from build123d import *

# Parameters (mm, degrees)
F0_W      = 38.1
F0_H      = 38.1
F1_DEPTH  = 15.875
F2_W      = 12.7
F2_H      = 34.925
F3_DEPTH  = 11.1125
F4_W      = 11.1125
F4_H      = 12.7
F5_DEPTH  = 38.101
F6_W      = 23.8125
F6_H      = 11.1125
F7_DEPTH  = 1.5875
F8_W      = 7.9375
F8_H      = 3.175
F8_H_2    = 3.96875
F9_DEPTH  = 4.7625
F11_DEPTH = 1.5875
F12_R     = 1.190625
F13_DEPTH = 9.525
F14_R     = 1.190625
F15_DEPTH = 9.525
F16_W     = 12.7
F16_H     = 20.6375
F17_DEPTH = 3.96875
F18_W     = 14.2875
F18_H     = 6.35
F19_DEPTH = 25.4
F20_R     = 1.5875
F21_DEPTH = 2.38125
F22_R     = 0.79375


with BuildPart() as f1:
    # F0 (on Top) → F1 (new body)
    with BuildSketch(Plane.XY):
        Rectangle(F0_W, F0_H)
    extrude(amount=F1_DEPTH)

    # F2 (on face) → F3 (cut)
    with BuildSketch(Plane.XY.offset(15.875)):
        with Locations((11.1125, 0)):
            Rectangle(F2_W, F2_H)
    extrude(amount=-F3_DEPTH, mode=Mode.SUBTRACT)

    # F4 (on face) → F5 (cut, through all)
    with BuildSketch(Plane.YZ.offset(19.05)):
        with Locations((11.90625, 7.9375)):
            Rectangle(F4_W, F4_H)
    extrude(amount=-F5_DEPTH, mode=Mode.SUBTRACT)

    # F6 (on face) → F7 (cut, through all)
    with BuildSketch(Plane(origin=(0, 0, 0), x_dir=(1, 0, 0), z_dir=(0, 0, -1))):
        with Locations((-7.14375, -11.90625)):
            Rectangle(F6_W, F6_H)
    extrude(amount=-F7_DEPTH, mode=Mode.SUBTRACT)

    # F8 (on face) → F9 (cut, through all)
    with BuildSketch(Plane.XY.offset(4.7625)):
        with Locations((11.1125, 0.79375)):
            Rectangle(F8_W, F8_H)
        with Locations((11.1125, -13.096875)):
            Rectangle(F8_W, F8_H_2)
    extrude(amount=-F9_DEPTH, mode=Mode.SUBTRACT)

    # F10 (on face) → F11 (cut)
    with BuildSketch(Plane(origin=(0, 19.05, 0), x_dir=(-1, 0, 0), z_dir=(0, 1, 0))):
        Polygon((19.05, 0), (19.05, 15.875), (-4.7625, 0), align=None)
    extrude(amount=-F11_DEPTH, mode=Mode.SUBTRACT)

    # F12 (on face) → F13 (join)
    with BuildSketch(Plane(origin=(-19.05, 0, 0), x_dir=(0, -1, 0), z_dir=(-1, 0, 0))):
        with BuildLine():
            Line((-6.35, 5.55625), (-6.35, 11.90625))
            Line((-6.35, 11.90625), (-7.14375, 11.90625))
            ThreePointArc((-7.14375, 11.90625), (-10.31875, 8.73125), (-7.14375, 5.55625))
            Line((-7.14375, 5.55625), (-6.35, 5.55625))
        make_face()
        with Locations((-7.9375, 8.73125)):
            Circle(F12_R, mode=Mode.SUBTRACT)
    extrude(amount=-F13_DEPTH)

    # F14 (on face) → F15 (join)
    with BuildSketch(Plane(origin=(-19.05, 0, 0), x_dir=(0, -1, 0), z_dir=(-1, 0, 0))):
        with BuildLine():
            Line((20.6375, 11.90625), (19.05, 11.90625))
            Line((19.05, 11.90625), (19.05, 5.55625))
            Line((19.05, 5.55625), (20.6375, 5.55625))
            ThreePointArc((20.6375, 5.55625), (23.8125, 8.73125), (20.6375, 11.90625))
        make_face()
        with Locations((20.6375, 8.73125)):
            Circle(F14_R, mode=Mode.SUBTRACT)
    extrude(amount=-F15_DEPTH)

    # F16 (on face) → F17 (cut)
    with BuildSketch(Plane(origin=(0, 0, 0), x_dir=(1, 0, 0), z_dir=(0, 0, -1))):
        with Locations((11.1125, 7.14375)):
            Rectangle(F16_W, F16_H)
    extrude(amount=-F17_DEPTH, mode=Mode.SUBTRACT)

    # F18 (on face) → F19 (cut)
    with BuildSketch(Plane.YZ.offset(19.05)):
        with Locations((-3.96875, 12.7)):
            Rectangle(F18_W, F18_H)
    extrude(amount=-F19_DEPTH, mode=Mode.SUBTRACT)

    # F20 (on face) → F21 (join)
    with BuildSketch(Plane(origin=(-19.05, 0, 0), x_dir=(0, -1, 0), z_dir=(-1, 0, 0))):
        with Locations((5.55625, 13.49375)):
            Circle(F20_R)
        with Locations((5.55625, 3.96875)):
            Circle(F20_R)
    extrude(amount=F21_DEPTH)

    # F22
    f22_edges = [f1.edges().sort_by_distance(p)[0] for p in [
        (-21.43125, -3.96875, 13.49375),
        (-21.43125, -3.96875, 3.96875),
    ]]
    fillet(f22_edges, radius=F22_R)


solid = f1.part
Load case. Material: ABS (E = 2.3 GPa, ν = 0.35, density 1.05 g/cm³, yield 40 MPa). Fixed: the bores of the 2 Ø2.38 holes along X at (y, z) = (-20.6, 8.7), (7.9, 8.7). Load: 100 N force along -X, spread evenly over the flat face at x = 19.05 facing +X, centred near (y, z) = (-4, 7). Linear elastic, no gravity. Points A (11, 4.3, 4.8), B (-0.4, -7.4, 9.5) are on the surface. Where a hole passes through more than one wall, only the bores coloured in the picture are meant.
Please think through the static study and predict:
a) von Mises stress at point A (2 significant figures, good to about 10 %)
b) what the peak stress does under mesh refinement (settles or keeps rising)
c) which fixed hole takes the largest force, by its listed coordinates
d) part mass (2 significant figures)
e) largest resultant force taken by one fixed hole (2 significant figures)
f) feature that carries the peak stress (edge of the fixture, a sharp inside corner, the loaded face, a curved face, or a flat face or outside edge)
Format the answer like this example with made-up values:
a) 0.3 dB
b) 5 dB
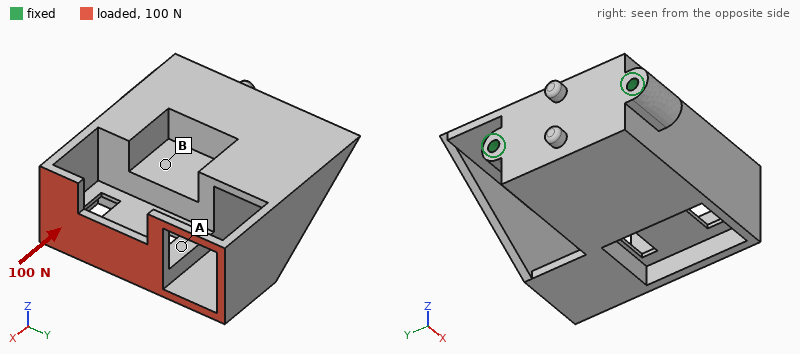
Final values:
a) 5.2 MPa
b) keeps rising
c) (7.9, 8.7)
d) 12 g
e) 61 N
f) a sharp inside corner
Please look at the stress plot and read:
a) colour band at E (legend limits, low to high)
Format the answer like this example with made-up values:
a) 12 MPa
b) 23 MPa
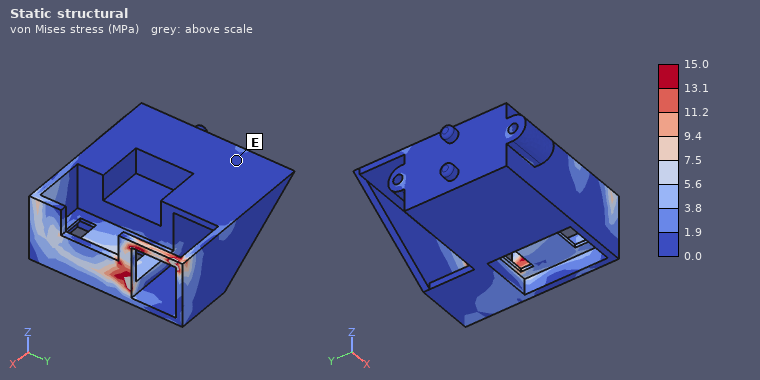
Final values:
a) 0.0 to 1.9 MPa
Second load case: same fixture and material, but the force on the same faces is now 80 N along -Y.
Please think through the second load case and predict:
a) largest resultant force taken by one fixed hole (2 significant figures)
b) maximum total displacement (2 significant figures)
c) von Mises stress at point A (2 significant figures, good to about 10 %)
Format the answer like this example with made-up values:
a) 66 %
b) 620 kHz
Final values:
a) 100 N
b) 0.40 mm
c) 5.6 MPa
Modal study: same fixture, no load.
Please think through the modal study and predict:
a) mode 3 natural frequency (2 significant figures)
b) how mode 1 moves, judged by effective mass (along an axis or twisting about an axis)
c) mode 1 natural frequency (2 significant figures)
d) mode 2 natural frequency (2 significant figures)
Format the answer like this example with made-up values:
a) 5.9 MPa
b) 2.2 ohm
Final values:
a) 2500 Hz
b) along Z
c) 1300 Hz
d) 2000 Hz
